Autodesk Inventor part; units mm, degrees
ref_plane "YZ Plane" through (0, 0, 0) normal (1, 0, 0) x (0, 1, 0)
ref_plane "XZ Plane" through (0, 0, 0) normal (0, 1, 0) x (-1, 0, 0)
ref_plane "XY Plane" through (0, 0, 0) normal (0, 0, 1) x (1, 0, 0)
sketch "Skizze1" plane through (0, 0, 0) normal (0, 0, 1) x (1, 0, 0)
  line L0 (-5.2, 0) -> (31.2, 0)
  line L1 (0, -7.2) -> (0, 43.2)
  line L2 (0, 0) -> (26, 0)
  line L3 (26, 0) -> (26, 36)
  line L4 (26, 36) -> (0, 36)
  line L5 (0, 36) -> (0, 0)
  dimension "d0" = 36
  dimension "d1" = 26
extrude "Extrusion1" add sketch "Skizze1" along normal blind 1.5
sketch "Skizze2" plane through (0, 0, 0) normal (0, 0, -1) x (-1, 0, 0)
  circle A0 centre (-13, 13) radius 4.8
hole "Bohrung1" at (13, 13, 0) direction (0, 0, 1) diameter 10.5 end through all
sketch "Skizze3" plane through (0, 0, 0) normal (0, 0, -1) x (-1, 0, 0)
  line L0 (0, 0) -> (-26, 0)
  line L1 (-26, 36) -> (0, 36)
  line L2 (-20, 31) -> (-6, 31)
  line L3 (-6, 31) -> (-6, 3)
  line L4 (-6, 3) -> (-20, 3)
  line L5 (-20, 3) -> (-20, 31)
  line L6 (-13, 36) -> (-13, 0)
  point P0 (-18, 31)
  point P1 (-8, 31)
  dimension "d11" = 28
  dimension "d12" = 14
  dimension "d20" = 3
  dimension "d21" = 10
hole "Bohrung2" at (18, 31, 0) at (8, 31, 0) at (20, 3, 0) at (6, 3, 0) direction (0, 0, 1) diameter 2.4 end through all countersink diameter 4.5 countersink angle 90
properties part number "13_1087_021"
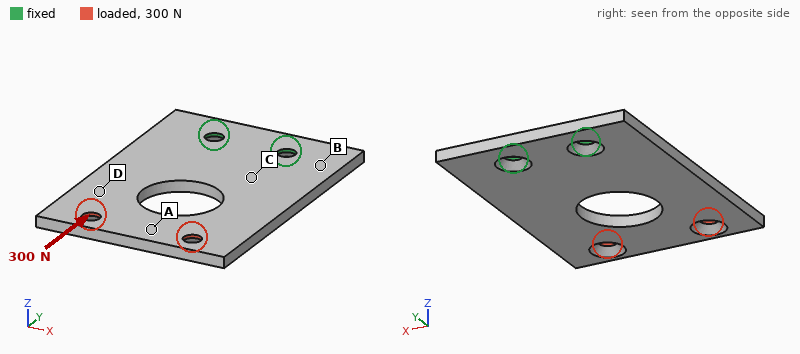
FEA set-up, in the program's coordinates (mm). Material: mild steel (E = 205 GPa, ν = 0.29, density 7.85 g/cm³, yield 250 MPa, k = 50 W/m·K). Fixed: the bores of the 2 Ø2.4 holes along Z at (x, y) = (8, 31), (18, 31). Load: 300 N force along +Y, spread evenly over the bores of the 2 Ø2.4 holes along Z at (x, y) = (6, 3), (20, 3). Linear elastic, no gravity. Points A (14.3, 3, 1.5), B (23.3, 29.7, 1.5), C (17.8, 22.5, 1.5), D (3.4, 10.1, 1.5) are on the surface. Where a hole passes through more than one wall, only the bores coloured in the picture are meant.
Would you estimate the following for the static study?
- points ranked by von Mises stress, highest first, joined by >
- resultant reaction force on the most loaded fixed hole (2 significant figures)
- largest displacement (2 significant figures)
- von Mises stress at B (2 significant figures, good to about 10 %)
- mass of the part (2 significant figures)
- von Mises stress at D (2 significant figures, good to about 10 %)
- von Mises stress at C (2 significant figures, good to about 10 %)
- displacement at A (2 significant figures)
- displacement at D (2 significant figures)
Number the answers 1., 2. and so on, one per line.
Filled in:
1. D > C > B > A
2. 150 N
3. 57 µm
4. 15 MPa
5. 9.6 g
6. 34 MPa
7. 25 MPa
8. 46 µm
9. 23 µm
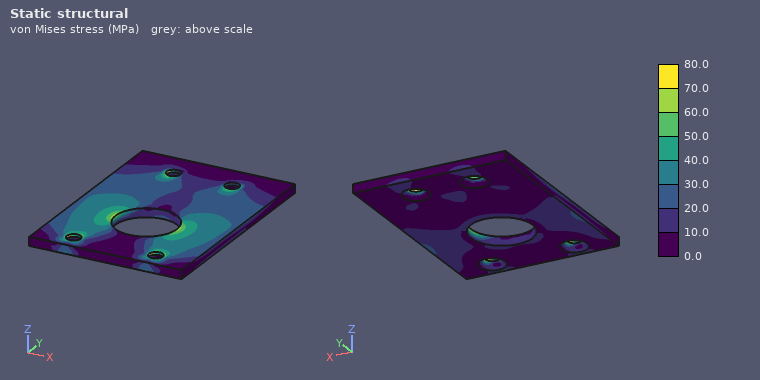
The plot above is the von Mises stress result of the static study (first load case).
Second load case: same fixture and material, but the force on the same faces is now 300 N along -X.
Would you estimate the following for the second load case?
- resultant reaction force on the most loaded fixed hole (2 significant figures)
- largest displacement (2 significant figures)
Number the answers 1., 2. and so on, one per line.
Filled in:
1. 740 N
2. 52 µm
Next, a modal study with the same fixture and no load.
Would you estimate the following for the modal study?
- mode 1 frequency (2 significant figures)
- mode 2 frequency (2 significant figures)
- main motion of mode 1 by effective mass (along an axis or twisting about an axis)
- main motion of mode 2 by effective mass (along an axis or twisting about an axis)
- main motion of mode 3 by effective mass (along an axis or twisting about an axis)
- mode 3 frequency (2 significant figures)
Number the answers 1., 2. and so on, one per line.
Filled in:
1. 1100 Hz
2. 3000 Hz
3. along Z
4. twisting about Y
5. along Z
6. 6400 Hz
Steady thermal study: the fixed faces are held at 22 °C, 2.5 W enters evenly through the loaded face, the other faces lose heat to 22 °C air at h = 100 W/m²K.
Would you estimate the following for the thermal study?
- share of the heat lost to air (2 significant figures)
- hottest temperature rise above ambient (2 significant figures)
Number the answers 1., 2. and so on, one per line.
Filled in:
1. 71 %
2. 28 K
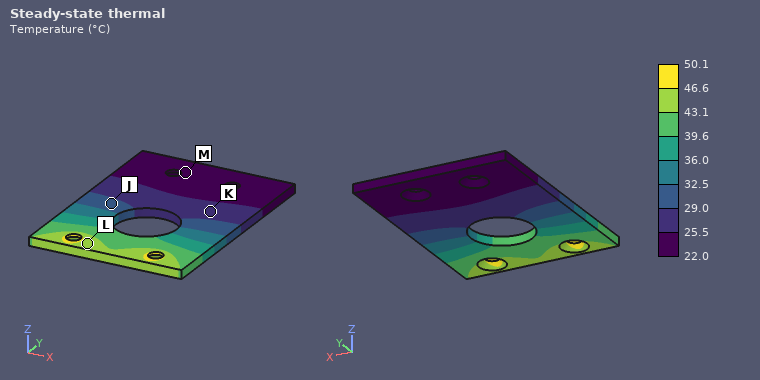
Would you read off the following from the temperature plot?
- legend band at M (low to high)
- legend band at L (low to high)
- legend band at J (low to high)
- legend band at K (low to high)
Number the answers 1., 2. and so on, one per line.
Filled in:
1. 22.0 to 25.5 °C
2. 43.1 to 46.6 °C
3. 29.0 to 32.5 °C
4. 25.5 to 29.0 °C
